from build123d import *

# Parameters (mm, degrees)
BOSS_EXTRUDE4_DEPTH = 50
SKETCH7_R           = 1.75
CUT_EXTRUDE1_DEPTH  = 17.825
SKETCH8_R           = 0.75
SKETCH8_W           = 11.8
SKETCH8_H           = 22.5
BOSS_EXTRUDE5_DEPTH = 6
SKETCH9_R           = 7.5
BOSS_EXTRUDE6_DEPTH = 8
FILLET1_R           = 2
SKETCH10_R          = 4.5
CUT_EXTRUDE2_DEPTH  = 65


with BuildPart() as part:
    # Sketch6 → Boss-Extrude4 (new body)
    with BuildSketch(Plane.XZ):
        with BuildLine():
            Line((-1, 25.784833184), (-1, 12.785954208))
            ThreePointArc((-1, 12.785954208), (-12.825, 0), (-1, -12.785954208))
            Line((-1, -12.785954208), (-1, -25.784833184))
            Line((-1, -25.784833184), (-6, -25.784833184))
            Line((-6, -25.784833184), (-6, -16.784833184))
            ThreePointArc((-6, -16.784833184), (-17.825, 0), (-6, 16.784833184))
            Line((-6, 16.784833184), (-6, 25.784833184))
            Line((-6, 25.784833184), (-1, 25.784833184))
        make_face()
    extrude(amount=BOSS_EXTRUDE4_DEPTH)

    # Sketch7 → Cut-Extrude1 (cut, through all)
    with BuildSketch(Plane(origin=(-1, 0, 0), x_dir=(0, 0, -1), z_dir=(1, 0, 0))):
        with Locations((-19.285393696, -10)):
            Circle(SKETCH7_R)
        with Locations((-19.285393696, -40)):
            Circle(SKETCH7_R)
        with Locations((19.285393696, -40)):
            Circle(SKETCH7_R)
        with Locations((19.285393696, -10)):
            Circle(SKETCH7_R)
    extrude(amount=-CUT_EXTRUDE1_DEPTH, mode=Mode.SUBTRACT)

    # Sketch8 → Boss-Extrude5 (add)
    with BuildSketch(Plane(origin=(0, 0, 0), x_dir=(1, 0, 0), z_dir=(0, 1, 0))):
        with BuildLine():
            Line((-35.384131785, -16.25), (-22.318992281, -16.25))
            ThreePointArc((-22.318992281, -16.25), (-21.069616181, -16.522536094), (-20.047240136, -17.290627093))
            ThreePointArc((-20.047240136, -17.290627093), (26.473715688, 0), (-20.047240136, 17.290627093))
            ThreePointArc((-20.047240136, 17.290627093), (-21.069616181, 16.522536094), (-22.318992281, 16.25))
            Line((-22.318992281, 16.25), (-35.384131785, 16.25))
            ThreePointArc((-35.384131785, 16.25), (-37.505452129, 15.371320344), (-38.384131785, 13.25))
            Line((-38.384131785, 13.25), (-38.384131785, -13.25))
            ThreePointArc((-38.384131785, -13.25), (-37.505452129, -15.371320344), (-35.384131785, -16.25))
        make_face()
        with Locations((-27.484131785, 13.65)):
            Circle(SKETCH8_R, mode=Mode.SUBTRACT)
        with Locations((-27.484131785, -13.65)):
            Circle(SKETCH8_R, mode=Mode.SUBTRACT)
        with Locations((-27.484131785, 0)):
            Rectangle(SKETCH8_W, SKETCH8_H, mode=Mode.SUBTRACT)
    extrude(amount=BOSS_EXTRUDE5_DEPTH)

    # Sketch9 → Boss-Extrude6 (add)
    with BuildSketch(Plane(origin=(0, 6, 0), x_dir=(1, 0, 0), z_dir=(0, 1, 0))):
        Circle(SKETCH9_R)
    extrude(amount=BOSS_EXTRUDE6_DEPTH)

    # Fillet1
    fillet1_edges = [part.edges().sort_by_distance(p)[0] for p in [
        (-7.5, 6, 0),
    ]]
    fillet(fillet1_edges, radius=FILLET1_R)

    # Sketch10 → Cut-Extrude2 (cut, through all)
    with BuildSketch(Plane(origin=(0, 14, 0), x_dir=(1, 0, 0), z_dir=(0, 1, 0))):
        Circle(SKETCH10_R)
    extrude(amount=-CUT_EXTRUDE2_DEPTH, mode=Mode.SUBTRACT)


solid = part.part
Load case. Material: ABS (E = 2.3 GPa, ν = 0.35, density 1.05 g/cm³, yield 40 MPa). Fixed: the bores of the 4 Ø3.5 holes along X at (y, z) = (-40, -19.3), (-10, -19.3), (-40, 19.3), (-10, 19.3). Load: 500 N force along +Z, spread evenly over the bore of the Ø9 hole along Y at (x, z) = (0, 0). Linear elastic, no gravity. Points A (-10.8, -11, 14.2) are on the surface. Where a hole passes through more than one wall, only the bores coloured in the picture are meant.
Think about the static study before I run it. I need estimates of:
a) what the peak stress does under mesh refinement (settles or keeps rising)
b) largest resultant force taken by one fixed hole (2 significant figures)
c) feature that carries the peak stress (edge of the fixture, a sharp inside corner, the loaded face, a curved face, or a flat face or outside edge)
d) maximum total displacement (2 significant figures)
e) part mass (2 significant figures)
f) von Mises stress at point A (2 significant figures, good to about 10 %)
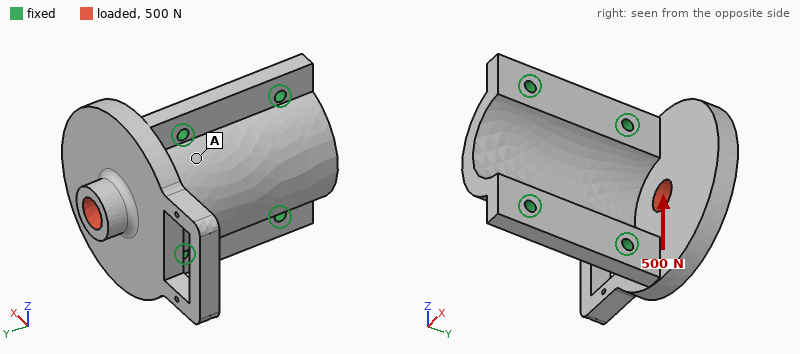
keeps rising
310 N
edge of the fixture
0.19 mm
32 g
2.2 MPa
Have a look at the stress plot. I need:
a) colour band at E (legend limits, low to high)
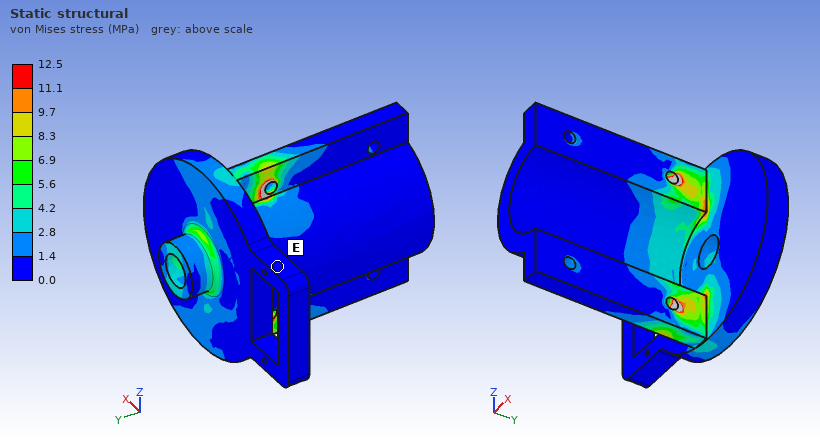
0.0 to 1.4 MPa
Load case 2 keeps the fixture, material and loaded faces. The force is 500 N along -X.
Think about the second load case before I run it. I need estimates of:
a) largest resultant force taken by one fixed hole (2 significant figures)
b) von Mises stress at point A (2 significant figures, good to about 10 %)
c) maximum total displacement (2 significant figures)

450 N
5.7 MPa
0.69 mm
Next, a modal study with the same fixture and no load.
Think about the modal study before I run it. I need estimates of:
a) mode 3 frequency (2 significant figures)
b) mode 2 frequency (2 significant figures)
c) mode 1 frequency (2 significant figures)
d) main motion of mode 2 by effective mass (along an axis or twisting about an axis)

2000 Hz
1700 Hz
1200 Hz
along Y
